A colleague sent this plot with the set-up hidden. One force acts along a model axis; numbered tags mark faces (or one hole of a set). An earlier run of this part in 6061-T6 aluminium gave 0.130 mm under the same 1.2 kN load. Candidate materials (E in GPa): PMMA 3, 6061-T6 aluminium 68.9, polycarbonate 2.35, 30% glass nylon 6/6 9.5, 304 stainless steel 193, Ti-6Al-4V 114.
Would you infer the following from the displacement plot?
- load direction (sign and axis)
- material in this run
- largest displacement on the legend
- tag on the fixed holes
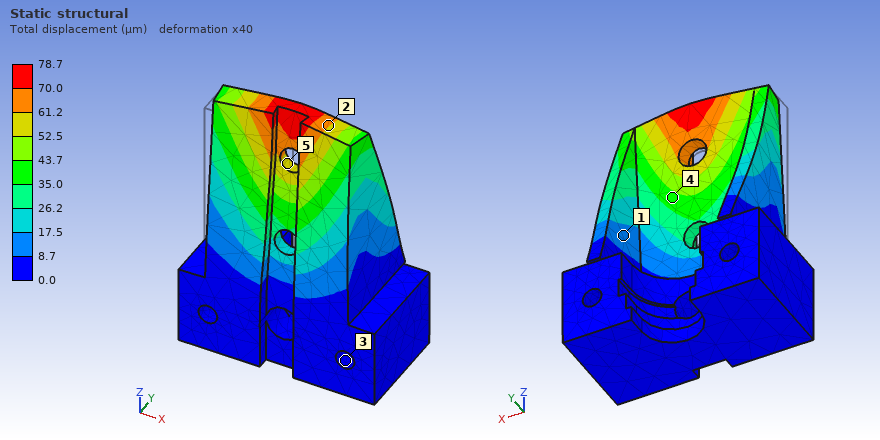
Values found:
+Y
Ti-6Al-4V
78.7 µm
3
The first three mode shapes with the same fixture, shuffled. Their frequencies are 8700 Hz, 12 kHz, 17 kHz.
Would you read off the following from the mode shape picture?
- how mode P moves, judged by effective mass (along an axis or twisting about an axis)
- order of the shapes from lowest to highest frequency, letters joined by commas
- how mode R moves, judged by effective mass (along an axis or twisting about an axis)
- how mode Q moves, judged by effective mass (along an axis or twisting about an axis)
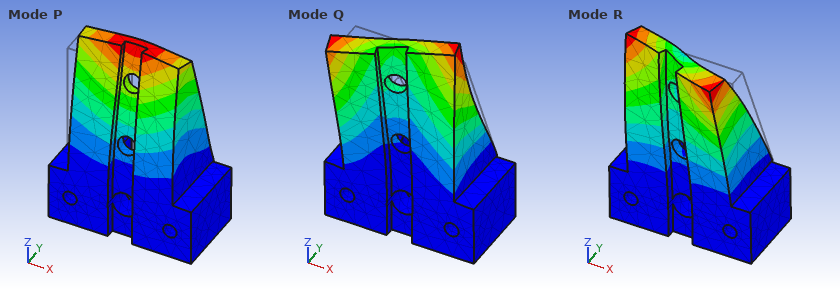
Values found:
along Y
P, Q, R
along X
along X
